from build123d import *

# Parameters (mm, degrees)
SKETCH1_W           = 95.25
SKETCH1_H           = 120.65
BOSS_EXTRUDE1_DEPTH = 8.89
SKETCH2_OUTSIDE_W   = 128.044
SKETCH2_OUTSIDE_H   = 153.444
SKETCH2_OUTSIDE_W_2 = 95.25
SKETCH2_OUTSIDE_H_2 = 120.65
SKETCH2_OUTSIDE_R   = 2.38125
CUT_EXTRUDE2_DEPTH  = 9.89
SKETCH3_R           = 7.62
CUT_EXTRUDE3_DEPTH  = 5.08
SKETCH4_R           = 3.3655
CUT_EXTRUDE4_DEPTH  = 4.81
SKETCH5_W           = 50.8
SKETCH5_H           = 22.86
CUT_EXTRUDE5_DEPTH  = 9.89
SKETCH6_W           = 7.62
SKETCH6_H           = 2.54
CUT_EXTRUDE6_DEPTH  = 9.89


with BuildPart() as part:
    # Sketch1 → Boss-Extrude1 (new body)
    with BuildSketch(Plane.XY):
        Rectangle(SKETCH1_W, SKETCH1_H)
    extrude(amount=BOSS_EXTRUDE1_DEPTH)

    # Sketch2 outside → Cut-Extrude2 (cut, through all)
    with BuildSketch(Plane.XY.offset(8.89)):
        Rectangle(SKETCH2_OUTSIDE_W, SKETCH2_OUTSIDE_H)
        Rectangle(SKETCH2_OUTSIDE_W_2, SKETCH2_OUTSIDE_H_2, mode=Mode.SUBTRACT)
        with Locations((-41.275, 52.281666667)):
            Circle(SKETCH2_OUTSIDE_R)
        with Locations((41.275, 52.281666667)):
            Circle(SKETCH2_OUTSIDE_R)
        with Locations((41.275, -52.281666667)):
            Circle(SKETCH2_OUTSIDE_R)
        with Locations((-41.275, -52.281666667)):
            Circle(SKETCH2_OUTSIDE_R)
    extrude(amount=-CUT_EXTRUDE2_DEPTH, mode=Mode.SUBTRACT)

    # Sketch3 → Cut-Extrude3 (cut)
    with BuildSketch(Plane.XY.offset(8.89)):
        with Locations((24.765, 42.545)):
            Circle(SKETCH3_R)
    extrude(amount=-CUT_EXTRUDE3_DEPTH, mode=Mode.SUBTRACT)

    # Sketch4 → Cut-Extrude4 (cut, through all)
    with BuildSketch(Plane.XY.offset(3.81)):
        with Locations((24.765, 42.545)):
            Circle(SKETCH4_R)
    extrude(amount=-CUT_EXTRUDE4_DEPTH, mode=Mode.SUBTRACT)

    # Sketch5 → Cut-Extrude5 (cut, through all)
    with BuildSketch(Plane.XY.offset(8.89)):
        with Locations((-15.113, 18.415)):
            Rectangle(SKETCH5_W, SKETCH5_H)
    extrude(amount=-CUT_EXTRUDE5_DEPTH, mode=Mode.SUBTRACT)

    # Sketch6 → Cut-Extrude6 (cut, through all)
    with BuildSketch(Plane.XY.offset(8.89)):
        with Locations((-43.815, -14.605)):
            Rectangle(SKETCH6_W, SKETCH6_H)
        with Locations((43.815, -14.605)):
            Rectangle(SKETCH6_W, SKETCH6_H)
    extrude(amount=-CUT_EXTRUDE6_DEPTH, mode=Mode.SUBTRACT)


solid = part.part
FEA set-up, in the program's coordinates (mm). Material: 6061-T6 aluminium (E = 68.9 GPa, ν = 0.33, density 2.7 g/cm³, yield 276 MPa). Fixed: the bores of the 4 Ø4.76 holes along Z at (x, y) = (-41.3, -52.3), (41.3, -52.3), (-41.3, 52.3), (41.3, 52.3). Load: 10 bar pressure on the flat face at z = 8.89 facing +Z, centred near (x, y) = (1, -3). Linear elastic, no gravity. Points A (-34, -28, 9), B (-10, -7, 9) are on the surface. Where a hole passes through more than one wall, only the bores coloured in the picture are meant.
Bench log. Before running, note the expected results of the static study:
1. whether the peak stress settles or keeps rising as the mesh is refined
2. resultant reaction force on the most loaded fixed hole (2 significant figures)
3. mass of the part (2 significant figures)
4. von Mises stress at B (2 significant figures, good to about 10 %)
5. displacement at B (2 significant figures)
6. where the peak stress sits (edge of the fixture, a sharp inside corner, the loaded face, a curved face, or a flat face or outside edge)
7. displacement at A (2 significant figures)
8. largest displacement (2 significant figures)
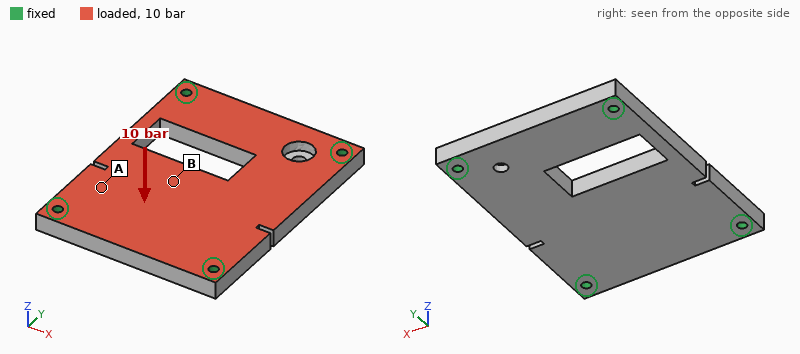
keeps rising
2.7 kN
240 g
31 MPa
0.20 mm
edge of the fixture
0.095 mm
0.23 mm
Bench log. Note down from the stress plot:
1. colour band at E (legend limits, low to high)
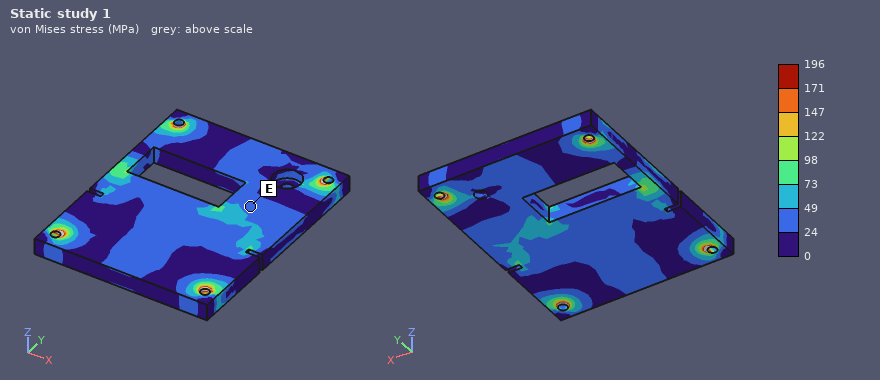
24 to 49 MPa
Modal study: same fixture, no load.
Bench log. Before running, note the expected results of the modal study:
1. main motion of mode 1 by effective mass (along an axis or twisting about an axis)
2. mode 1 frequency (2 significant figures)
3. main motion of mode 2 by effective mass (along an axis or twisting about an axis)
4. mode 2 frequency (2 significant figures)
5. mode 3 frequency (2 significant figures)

along Z
2800 Hz
twisting about Y
4500 Hz
5800 Hz
